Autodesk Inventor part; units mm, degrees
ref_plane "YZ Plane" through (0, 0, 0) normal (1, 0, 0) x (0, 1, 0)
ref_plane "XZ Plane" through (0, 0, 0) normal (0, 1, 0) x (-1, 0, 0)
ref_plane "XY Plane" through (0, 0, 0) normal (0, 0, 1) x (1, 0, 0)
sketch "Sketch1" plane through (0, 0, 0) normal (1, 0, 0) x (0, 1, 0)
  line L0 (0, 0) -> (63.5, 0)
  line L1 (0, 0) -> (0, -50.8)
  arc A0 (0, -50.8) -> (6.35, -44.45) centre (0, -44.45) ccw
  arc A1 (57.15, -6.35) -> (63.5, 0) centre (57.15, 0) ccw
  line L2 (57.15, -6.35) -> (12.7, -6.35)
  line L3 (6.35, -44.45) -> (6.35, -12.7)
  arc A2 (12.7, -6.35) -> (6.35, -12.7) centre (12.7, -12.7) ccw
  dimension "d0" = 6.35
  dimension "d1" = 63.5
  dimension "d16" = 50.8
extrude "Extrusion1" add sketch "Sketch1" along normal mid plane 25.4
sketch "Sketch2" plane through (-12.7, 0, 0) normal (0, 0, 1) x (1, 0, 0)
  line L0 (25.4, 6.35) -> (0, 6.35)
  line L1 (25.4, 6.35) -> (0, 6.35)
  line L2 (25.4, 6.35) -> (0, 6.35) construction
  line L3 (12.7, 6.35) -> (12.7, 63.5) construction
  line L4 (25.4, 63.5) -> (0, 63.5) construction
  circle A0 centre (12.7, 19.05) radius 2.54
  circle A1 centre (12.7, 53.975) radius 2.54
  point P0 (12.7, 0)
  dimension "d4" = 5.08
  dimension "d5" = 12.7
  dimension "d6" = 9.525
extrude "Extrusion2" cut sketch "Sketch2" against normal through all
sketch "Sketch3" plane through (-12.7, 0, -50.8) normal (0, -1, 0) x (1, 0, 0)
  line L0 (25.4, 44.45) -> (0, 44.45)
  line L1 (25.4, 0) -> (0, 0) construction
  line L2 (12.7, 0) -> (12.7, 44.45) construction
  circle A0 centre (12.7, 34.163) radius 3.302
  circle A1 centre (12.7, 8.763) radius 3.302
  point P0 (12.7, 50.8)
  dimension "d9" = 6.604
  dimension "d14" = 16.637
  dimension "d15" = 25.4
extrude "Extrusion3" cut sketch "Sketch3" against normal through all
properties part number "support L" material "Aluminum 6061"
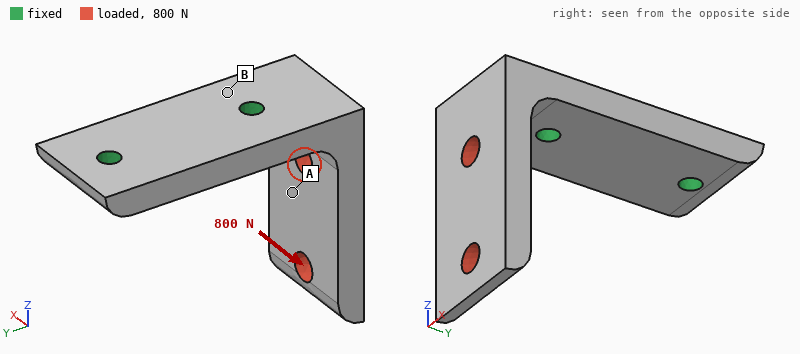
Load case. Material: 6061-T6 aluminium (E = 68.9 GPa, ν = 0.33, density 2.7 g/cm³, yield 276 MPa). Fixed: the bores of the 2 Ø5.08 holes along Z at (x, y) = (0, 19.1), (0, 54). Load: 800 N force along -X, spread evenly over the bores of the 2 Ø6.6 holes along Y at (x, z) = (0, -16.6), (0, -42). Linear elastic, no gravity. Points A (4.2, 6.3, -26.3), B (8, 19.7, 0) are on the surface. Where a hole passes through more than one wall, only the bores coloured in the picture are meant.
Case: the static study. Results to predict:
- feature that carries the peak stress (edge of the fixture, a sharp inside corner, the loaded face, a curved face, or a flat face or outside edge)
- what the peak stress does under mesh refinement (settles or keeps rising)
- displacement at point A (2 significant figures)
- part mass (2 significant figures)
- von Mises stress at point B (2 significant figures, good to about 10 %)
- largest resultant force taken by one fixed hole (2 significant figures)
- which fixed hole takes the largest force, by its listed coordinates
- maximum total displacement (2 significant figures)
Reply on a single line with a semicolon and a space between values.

edge of the fixture; keeps rising; 0.12 mm; 45 g; 55 MPa; 1.1 kN; (0, 19.1); 0.24 mm
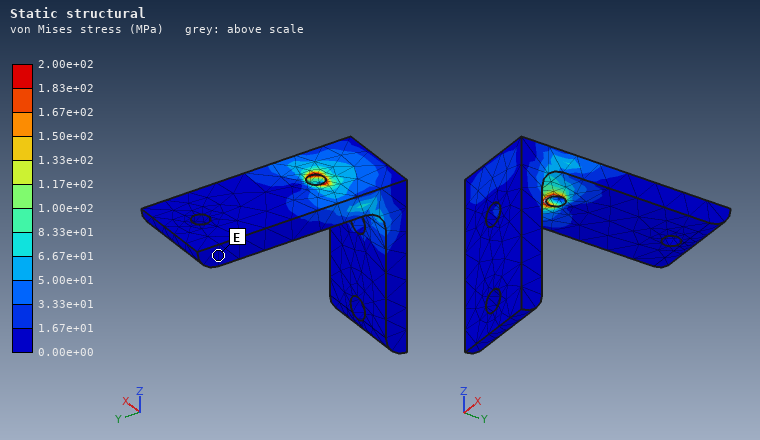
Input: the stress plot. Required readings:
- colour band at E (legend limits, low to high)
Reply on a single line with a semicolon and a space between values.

0.00e+00 to 1.67e+01 MPa
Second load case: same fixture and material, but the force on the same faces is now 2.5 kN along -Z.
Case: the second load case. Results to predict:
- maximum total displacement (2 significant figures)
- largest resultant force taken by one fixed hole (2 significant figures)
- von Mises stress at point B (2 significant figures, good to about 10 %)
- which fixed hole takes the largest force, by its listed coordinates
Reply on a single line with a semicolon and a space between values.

0.41 mm; 2.7 kN; 87 MPa; (0, 19.1)
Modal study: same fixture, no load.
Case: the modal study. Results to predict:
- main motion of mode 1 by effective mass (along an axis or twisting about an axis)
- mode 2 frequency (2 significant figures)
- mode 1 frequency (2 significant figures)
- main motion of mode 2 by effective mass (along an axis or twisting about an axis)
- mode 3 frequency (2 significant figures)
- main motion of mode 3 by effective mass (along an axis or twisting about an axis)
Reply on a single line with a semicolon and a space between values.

along Y; 2700 Hz; 1800 Hz; along X; 6900 Hz; along Z
